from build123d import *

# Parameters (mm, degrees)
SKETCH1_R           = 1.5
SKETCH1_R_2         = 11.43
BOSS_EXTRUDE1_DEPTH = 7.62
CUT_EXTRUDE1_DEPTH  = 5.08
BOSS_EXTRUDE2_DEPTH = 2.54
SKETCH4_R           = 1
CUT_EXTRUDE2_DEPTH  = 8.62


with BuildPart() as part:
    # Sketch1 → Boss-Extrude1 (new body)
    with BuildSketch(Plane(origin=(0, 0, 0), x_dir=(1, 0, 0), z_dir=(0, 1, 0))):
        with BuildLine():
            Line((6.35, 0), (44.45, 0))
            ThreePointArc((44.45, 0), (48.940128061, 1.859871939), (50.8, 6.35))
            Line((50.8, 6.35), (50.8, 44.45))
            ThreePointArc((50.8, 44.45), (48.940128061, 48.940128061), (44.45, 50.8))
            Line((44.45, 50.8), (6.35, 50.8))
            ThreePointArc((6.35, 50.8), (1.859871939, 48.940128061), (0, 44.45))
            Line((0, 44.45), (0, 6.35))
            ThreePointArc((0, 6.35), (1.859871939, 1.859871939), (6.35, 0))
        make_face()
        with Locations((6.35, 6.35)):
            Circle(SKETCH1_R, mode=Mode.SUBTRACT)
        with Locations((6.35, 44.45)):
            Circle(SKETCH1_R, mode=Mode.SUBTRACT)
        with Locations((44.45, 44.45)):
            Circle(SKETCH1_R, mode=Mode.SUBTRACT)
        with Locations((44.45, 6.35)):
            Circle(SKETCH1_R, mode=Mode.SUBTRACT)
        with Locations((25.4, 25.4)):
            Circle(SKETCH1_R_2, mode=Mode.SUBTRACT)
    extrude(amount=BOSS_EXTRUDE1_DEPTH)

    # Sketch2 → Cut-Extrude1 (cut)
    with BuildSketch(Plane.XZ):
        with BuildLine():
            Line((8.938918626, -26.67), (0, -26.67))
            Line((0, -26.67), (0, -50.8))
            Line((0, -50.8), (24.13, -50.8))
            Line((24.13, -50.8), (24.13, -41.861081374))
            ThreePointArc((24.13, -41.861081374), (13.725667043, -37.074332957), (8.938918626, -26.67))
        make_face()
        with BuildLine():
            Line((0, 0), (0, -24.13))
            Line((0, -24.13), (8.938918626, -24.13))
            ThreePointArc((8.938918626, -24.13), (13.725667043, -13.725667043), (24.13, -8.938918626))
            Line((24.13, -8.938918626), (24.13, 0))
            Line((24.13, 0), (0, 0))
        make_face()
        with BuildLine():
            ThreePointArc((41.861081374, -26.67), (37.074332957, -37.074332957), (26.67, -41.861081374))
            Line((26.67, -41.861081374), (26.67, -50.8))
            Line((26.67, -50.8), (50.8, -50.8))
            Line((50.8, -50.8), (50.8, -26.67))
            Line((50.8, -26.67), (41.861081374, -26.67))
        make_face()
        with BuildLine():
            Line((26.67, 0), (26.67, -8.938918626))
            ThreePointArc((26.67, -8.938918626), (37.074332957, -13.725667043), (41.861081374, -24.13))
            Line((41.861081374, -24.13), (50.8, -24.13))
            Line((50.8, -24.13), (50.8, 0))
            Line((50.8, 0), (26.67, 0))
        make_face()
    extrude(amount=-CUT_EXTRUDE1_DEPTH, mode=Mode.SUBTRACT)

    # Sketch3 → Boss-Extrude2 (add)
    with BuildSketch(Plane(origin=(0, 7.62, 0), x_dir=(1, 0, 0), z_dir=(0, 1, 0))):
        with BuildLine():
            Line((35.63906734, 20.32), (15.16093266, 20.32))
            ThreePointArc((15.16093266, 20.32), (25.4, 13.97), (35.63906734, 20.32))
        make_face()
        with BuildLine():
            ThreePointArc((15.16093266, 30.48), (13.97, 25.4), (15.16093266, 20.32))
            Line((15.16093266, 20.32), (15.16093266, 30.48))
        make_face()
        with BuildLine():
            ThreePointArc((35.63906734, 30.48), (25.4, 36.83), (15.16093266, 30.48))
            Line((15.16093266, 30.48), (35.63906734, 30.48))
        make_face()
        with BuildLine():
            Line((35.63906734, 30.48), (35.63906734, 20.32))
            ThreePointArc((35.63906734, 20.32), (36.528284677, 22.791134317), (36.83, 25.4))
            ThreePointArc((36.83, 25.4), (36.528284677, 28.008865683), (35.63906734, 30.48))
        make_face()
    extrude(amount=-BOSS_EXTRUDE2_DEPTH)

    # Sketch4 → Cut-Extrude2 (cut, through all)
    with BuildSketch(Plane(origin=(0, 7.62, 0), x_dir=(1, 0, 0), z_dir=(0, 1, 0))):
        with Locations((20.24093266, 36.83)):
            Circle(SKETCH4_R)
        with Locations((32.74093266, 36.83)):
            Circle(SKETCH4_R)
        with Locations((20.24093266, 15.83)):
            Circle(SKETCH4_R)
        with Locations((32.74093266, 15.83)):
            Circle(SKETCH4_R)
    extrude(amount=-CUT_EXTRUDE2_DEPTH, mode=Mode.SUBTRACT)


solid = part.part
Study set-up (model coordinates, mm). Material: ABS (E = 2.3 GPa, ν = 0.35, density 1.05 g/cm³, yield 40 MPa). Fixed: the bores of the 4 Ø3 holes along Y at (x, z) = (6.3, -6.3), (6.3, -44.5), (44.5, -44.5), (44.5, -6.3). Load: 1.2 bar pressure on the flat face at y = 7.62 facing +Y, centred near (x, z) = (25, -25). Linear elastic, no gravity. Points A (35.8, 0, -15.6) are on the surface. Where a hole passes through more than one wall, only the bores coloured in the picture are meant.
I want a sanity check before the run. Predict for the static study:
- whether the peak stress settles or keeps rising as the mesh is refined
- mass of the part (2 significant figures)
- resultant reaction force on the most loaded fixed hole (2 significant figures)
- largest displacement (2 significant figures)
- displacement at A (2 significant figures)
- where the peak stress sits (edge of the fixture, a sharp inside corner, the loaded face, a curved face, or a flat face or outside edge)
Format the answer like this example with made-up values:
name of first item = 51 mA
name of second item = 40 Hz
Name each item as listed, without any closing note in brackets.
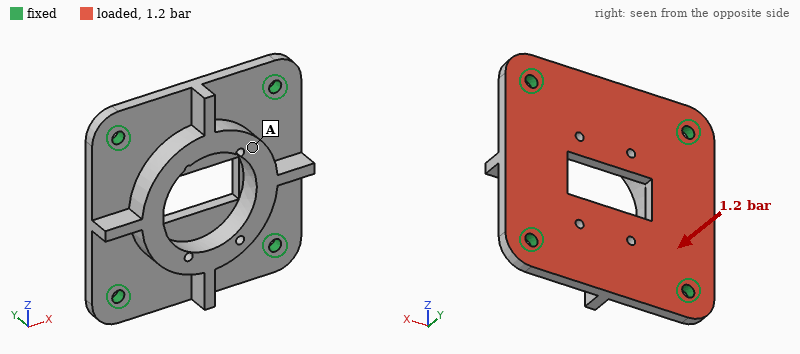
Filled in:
whether the peak stress settles or keeps rising as the mesh is refined = keeps rising
mass of the part = 8.9 g
resultant reaction force on the most loaded fixed hole = 72 N
largest displacement = 0.18 mm
displacement at A = 0.15 mm
where the peak stress sits = edge of the fixture
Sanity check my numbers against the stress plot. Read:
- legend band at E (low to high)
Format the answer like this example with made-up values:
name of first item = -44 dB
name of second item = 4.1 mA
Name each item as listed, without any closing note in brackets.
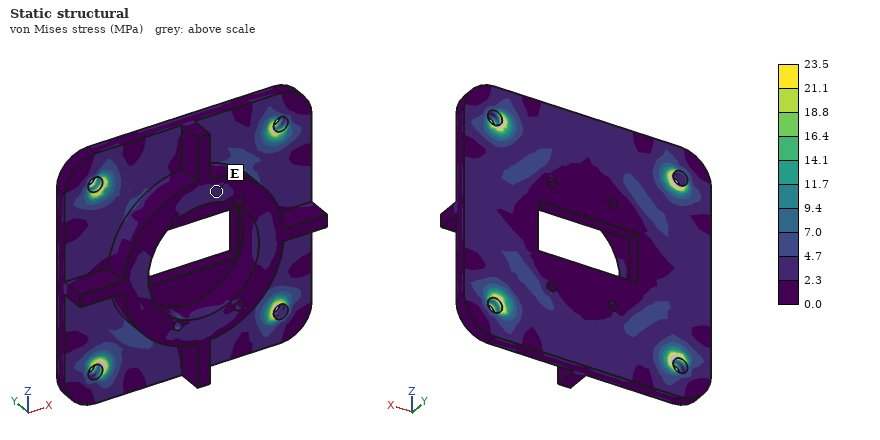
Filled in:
legend band at E = 2.3 to 4.7 MPa
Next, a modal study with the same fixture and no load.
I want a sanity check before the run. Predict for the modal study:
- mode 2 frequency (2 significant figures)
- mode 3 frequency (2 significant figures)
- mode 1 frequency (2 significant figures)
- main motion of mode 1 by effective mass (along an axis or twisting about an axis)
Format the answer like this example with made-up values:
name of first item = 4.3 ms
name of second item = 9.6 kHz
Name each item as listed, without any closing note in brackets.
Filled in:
mode 2 frequency = 2800 Hz
mode 3 frequency = 2900 Hz
mode 1 frequency = 2200 Hz
main motion of mode 1 by effective mass = along Y
